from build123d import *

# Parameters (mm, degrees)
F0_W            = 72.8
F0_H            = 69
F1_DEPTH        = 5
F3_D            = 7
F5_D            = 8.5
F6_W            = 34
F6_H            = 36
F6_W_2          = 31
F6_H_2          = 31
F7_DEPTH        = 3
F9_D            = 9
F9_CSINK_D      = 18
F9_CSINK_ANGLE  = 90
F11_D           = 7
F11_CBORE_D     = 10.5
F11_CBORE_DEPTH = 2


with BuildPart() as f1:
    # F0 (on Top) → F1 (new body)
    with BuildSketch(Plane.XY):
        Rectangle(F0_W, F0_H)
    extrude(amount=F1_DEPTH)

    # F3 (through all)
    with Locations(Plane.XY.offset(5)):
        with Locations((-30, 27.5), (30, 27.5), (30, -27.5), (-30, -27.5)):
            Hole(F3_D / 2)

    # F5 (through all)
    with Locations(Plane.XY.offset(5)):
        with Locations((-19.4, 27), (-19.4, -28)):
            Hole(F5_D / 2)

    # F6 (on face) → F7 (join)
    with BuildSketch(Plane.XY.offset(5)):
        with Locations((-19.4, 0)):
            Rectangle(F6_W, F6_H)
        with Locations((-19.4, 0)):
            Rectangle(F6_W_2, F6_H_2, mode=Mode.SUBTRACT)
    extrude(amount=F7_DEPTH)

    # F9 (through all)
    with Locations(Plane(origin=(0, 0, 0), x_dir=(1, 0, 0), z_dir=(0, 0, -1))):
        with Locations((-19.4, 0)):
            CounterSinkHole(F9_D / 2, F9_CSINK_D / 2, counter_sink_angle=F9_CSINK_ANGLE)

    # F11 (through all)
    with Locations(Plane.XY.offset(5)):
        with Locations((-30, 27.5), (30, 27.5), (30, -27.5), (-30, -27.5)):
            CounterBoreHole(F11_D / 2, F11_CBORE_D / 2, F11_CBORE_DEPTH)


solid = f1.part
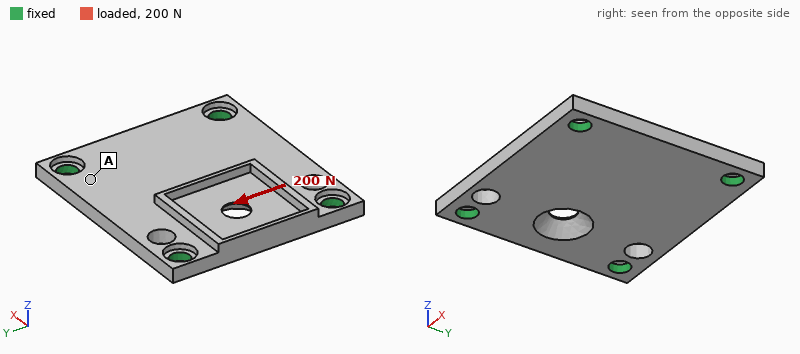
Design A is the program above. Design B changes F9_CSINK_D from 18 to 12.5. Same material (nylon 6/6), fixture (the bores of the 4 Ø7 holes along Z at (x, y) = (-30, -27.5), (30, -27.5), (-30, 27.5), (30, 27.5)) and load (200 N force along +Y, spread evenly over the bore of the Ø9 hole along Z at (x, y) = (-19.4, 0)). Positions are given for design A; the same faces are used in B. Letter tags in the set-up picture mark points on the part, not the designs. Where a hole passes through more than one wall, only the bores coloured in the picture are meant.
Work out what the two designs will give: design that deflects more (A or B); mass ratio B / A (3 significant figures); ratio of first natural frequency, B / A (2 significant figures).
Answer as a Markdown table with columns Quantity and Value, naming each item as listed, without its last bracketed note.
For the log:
| Quantity | Value |
|---|---|
| design that deflects more | A |
| mass ratio B / A | 1.01 |
| ratio of first natural frequency, B / A | 1.00 |
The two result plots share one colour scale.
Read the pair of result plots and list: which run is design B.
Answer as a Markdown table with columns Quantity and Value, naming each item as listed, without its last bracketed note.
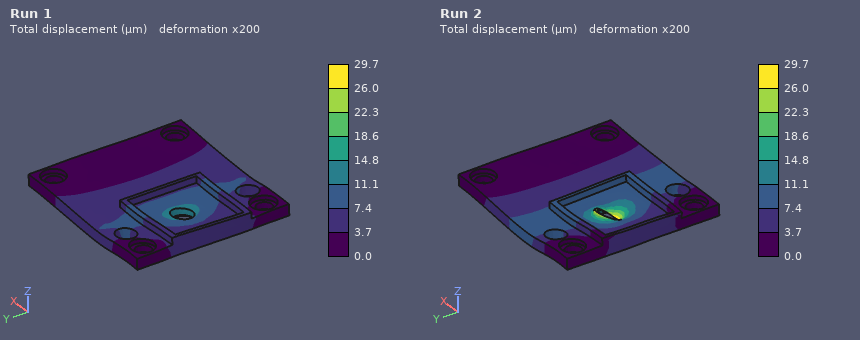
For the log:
| Quantity | Value |
|---|---|
| which run is design B | Run 1 |
